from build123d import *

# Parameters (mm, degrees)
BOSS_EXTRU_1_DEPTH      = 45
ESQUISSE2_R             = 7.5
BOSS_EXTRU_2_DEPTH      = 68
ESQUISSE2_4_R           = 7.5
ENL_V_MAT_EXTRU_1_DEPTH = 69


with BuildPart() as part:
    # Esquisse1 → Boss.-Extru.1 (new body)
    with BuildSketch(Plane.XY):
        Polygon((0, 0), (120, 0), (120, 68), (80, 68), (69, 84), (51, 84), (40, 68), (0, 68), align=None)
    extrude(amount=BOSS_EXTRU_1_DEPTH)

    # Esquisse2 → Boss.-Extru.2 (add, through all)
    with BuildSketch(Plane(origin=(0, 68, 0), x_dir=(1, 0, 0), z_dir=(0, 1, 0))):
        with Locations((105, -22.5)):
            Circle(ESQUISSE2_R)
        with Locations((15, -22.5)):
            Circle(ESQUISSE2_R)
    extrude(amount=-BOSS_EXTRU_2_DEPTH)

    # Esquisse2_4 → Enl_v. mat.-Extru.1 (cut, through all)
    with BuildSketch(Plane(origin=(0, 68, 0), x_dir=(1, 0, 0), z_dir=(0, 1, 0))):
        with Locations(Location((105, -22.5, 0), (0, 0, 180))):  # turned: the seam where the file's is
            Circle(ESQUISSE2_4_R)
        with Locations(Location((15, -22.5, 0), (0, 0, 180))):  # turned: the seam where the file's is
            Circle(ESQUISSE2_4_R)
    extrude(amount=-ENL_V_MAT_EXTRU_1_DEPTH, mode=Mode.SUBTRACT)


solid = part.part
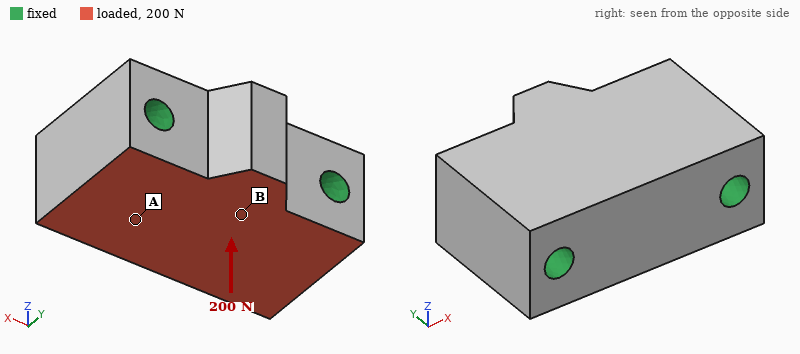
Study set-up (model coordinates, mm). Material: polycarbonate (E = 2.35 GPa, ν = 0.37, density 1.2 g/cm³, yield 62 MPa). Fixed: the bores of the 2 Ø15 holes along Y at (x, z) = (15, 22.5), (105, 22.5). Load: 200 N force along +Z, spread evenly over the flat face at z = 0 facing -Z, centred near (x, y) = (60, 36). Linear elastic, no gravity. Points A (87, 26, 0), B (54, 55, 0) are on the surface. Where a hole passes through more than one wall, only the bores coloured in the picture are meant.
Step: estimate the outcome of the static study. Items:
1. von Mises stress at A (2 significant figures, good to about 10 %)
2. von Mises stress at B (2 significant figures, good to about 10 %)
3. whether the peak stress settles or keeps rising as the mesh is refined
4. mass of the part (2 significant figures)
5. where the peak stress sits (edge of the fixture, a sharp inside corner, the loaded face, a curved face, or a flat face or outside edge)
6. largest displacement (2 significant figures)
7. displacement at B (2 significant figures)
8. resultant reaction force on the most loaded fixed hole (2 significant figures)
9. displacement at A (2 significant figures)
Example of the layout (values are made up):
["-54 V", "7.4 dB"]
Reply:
["0.022 MPa", "0.051 MPa", "keeps rising", "440 g", "edge of the fixture", "2.1 µm", "1.3 µm", "100 N", "0.69 µm"]
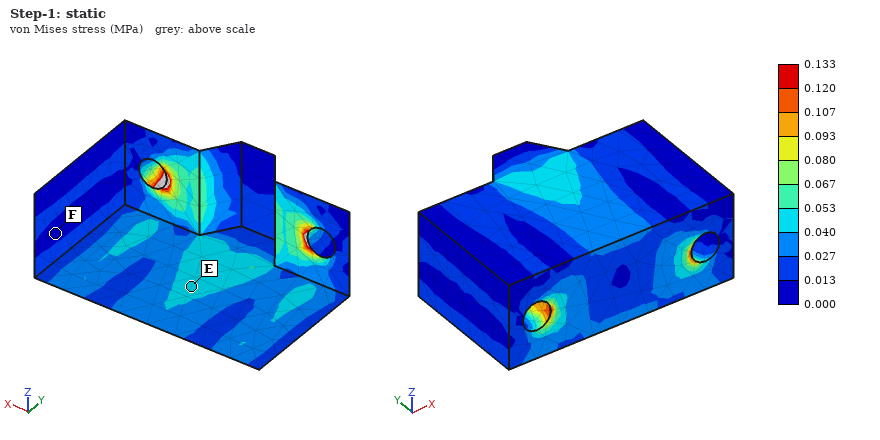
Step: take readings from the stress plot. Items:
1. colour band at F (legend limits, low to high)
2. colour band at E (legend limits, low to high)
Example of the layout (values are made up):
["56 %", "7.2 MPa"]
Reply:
["0.000 to 0.013 MPa", "0.040 to 0.053 MPa"]
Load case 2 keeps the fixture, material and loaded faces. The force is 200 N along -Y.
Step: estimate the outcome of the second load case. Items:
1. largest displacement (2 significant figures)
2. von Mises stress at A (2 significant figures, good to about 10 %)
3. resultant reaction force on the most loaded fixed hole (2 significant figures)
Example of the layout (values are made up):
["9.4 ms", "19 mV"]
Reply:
["3.2 µm", "0.075 MPa", "100 N"]
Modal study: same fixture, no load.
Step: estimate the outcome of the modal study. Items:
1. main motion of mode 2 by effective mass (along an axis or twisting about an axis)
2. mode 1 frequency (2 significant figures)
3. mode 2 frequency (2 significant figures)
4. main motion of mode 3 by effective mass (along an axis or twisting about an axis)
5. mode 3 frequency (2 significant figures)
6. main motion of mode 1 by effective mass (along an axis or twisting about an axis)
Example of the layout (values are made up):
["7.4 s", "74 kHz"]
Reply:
["along Z", "3100 Hz", "3900 Hz", "along Y", "4100 Hz", "along Z"]
